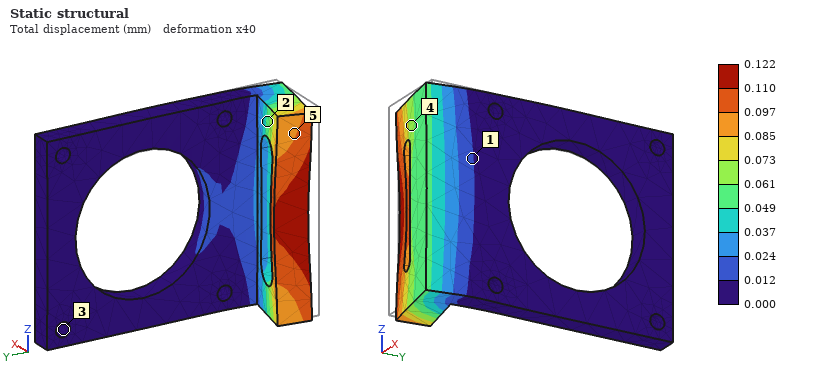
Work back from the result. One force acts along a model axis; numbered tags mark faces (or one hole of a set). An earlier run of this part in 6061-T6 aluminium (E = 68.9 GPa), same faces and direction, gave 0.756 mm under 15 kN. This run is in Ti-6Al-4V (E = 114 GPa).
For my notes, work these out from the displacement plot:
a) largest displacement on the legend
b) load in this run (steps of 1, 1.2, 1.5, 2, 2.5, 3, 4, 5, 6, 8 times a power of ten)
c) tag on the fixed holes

0.122 mm
4 kN
3
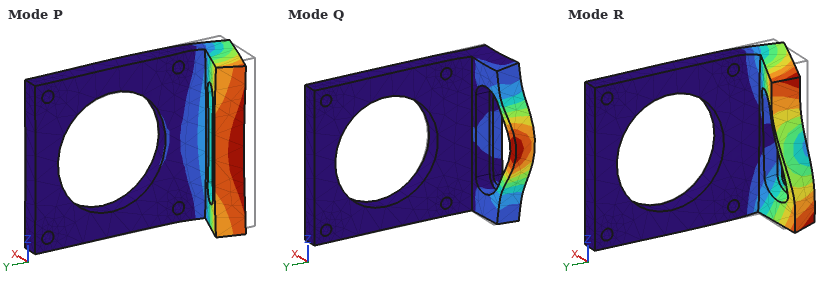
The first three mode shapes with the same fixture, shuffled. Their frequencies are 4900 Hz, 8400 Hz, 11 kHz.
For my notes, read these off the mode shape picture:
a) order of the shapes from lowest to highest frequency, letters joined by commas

P, R, Q
